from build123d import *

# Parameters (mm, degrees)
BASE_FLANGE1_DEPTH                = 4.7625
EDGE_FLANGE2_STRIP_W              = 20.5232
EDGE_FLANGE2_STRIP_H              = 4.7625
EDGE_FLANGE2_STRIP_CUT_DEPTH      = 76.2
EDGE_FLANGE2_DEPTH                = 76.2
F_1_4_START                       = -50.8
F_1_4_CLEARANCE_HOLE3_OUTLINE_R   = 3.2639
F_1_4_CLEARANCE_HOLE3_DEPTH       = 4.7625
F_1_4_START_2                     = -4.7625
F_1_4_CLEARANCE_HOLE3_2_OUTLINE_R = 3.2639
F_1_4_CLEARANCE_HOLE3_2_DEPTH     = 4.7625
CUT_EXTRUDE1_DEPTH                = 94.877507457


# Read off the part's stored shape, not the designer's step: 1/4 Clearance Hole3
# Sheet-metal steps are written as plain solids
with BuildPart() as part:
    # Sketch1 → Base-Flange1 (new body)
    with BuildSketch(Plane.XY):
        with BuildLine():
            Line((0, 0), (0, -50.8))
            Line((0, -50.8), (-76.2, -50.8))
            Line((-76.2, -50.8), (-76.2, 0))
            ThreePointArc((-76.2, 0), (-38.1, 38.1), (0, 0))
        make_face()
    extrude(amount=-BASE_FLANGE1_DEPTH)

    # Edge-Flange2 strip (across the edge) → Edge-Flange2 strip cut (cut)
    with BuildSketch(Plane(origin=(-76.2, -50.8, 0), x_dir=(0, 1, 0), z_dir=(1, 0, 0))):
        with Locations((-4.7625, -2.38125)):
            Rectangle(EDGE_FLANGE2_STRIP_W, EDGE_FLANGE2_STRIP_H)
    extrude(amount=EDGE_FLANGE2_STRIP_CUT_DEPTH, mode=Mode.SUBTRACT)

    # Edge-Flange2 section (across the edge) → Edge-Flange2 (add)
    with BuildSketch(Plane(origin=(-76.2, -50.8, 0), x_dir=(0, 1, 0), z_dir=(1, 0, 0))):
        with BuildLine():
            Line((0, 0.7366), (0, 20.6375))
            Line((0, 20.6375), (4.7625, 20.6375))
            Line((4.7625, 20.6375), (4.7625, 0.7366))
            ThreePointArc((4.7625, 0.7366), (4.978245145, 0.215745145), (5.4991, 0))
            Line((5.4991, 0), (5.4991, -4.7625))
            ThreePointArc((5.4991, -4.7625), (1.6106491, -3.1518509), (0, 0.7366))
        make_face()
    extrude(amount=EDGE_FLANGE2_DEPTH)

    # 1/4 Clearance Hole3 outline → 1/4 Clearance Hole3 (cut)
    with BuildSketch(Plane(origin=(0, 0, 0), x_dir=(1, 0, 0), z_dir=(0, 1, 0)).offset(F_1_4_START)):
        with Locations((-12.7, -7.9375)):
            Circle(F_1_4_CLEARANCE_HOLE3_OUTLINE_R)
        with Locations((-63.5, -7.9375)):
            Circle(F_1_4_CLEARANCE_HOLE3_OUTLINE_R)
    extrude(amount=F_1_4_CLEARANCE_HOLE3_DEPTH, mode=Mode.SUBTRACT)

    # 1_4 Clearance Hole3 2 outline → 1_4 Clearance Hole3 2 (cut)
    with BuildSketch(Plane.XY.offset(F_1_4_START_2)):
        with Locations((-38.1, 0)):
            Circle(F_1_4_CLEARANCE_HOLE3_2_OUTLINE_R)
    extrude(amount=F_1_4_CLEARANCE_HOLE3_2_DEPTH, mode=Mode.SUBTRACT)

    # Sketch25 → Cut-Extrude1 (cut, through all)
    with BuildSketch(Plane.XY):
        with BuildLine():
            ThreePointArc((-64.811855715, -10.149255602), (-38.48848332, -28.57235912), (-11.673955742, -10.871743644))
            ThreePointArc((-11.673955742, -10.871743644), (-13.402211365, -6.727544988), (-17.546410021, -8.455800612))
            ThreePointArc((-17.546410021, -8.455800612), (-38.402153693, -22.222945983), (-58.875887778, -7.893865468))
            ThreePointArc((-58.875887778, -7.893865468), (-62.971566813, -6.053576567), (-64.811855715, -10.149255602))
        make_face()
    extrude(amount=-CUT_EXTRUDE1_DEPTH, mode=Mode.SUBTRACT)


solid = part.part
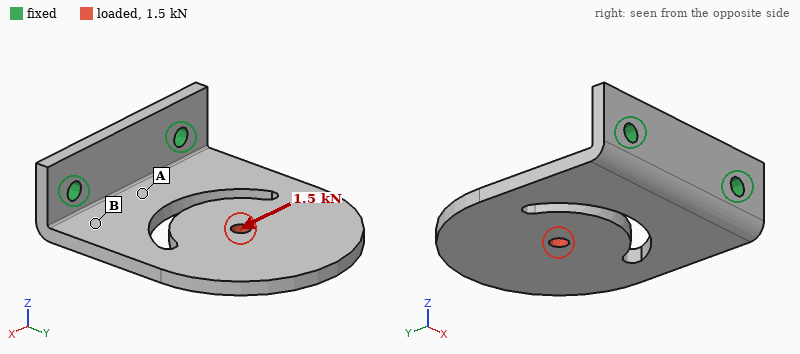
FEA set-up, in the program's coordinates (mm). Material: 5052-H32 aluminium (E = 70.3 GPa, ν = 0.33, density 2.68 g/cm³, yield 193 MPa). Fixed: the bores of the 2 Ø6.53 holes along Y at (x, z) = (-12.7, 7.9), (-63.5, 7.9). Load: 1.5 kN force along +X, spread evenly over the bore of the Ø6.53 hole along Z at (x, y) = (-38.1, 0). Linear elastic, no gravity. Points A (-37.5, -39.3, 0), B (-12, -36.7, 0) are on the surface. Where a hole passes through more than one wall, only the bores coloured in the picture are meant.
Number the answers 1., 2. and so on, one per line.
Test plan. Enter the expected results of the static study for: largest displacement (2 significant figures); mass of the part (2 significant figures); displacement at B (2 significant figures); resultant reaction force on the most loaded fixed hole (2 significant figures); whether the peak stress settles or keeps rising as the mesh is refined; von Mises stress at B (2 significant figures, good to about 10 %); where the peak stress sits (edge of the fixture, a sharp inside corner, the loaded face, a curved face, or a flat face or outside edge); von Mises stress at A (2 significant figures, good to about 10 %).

1. 0.14 mm
2. 91 g
3. 0.033 mm
4. 1.6 kN
5. keeps rising
6. 19 MPa
7. edge of the fixture
8. 39 MPa
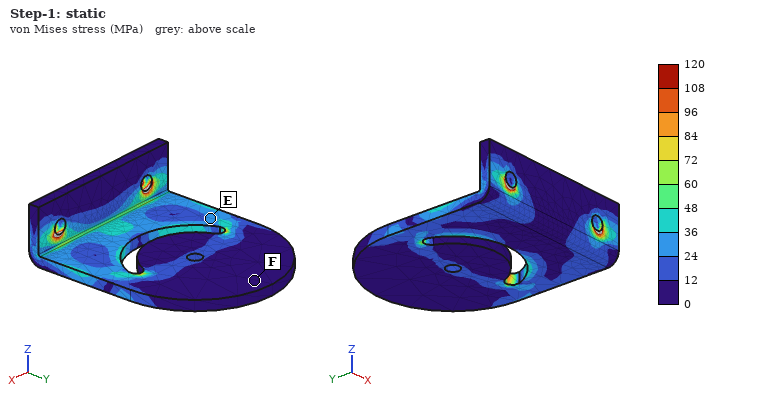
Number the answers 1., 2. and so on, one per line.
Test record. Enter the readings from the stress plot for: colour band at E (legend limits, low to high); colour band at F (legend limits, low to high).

1. 24 to 36 MPa
2. 0 to 12 MPa
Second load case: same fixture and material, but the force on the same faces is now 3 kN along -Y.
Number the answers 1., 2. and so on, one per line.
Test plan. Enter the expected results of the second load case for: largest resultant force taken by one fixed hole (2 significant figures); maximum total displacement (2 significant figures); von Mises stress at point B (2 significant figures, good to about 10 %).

1. 1.5 kN
2. 0.31 mm
3. 19 MPa
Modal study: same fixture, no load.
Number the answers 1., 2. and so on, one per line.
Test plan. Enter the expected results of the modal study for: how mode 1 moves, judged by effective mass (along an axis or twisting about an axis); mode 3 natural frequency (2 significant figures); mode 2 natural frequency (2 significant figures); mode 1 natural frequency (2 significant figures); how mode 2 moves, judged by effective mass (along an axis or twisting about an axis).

1. along Z
2. 2100 Hz
3. 1500 Hz
4. 440 Hz
5. twisting about Y
